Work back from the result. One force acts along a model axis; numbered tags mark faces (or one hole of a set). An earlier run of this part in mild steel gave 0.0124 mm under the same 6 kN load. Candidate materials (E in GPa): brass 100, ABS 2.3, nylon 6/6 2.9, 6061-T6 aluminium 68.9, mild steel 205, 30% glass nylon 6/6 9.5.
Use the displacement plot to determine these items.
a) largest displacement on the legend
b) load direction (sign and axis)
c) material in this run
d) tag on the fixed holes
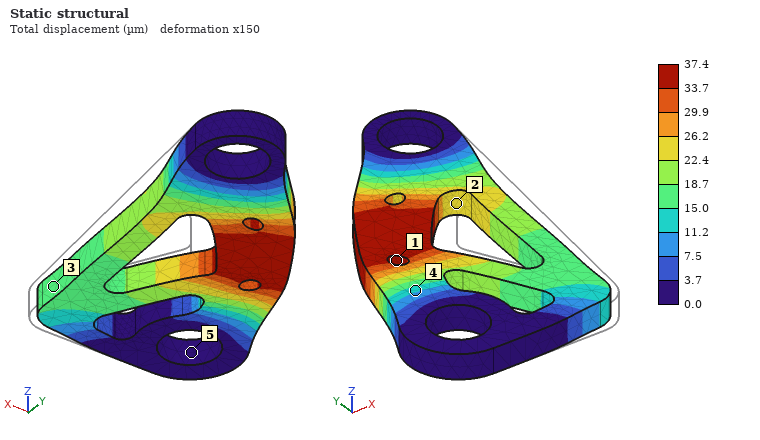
37.4 µm
-X
6061-T6 aluminium
5
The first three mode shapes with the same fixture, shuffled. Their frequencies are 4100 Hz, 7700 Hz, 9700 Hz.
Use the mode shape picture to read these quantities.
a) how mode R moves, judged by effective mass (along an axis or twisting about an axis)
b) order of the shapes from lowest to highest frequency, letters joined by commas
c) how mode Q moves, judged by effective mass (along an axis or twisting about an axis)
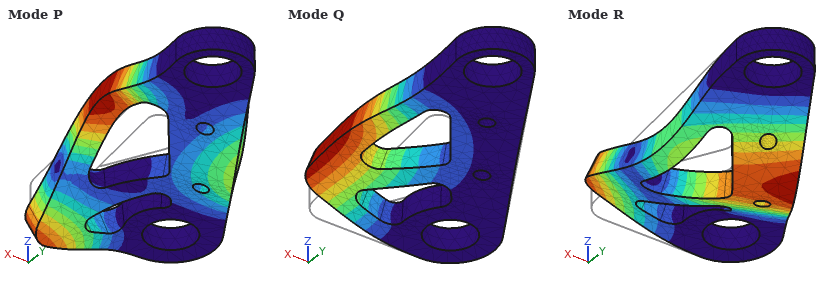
along Z
Q, R, P
along Z
